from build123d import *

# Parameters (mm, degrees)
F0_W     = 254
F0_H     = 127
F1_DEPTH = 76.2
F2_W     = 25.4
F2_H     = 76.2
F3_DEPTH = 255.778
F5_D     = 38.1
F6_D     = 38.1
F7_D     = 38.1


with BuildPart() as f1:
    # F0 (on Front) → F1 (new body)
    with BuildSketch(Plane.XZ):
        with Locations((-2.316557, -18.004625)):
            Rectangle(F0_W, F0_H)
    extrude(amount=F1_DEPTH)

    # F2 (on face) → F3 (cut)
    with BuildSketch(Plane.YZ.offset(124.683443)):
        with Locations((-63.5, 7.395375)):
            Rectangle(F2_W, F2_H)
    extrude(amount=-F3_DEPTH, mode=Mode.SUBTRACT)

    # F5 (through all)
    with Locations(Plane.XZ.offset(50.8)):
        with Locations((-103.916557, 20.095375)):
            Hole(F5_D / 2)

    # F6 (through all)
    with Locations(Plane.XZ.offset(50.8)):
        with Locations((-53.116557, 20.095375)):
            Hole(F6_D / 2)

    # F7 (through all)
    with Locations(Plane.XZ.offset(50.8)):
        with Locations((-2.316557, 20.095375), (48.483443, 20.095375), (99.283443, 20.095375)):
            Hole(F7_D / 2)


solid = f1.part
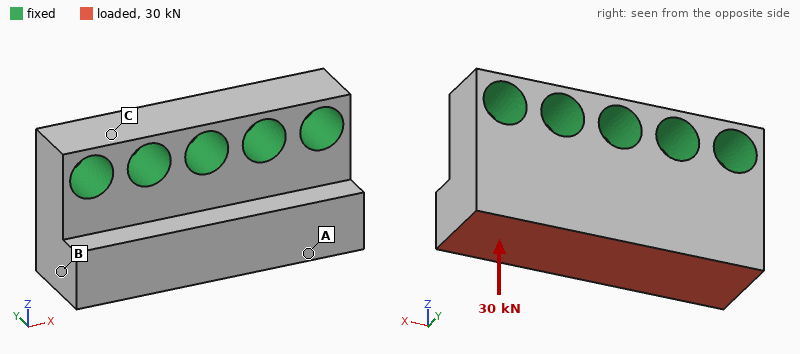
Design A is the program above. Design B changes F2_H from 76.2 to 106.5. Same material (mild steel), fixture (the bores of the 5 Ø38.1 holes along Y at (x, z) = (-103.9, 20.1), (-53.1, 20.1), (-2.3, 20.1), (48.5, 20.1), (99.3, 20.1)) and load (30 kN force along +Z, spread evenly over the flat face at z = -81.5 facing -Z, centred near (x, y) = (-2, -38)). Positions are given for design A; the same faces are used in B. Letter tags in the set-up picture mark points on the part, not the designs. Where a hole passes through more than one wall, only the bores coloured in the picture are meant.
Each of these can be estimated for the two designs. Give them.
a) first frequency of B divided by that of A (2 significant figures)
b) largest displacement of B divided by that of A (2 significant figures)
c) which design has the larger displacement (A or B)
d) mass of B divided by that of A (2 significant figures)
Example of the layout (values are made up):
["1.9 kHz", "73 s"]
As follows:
["1.0", "1.2", "B", "0.94"]
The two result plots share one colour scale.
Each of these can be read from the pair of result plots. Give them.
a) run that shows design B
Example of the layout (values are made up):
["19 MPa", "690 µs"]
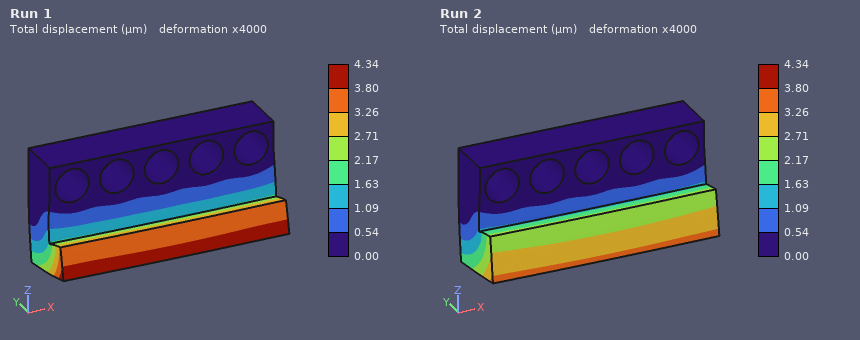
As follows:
["Run 1"]
